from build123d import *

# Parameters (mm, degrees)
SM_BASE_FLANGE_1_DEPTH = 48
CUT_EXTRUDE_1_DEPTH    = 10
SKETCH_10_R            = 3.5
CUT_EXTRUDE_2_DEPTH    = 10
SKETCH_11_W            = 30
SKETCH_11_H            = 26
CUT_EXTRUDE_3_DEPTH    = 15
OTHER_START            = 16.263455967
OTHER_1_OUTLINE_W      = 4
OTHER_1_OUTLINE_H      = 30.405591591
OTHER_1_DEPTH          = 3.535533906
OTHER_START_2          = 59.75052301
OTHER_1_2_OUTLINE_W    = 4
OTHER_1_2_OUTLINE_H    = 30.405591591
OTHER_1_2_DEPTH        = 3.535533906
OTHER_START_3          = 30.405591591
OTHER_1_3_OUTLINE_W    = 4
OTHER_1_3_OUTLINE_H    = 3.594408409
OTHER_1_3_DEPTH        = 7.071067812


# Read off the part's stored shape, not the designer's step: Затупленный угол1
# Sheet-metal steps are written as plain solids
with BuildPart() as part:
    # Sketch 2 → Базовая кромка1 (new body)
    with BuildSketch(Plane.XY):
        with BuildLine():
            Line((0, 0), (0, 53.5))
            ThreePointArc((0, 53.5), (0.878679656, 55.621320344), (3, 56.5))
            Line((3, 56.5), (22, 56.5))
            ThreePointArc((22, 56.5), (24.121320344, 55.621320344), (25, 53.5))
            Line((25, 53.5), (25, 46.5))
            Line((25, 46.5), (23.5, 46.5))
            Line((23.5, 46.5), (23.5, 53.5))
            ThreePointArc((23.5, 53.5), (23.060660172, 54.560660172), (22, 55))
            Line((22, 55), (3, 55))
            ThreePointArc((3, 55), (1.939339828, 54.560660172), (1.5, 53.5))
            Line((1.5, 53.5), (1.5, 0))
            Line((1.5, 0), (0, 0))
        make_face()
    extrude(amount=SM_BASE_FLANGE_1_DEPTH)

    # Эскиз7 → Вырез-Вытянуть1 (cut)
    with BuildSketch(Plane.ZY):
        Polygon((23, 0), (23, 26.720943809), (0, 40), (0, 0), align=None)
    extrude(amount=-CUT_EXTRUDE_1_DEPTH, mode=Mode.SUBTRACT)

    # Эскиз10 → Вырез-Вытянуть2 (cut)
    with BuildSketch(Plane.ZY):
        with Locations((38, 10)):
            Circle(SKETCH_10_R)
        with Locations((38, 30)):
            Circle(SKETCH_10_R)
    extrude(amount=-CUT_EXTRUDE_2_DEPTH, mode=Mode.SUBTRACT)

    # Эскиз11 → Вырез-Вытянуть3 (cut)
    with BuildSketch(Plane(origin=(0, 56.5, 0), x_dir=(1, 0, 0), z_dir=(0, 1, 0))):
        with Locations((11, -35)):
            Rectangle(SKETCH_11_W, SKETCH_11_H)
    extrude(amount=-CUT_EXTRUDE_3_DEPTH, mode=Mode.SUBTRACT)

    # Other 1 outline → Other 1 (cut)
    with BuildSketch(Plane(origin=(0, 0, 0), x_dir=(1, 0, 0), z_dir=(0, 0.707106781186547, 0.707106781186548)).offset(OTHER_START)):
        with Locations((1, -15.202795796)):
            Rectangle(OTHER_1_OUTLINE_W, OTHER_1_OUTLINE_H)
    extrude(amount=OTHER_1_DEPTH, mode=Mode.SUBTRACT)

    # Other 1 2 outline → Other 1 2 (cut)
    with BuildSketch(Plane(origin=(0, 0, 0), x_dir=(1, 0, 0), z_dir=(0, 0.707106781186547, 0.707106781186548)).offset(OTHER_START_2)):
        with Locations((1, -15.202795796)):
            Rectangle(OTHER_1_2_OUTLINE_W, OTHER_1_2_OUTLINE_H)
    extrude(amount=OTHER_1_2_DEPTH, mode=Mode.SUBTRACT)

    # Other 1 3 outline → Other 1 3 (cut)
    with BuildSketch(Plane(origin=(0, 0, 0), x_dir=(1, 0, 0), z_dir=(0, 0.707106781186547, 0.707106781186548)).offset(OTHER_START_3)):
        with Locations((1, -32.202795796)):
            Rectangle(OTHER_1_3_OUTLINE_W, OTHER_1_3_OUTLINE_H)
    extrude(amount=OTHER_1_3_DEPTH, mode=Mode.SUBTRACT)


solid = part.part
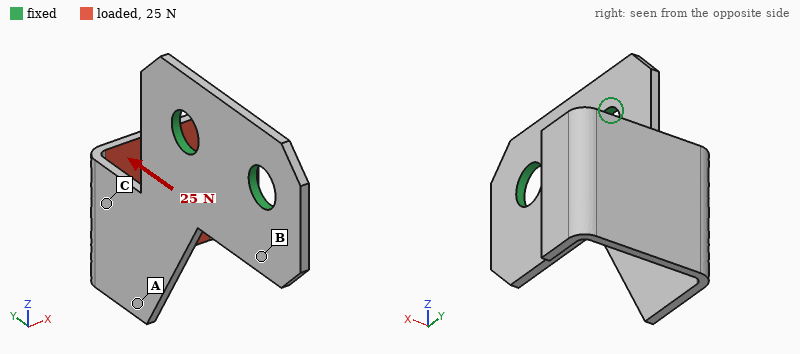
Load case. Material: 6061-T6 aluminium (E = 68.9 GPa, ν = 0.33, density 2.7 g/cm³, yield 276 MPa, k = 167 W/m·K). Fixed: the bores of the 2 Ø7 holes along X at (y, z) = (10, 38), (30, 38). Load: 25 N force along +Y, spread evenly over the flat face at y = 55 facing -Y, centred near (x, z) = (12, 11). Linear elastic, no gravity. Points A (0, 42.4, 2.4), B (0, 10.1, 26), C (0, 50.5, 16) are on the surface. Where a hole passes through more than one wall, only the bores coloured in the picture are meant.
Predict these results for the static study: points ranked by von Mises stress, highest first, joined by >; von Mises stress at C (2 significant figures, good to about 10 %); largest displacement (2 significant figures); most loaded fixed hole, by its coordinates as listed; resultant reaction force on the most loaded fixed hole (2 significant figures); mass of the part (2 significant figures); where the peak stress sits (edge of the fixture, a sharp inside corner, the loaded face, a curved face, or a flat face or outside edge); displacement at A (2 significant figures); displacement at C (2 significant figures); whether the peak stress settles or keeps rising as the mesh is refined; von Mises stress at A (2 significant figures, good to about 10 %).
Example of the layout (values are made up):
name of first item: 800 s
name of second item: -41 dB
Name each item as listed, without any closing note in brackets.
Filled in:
points ranked by von Mises stress, highest first, joined by >: C > A > B
von Mises stress at C: 34 MPa
largest displacement: 0.83 mm
most loaded fixed hole, by its coordinates as listed: (10, 38)
resultant reaction force on the most loaded fixed hole: 29 N
mass of the part: 8.5 g
where the peak stress sits: a sharp inside corner
displacement at A: 0.16 mm
displacement at C: 0.28 mm
whether the peak stress settles or keeps rising as the mesh is refined: keeps rising
von Mises stress at A: 22 MPa
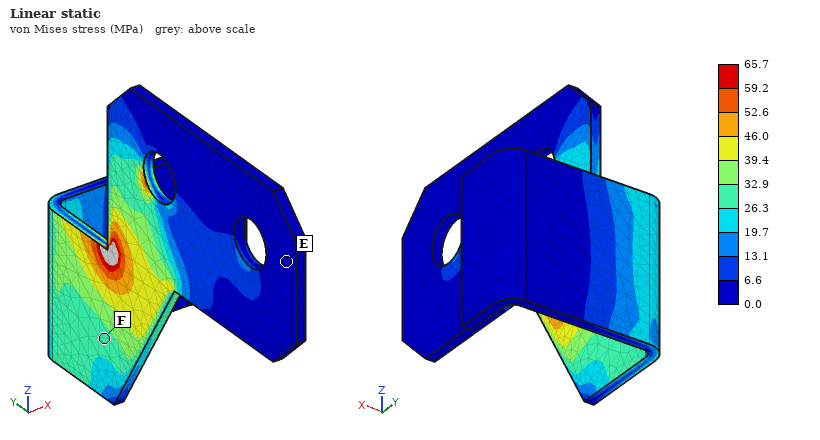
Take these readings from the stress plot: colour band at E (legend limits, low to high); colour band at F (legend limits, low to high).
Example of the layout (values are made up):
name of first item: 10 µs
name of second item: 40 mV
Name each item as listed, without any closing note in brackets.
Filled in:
colour band at E: 0.0 to 6.6 MPa
colour band at F: 26.3 to 32.9 MPa
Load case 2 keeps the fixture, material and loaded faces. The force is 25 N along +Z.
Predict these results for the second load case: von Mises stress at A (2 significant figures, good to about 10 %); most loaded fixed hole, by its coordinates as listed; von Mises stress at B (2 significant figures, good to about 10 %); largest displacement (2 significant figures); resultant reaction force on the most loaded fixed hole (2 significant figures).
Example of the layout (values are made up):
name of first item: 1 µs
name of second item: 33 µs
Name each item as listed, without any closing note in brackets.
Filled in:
von Mises stress at A: 11 MPa
most loaded fixed hole, by its coordinates as listed: (30, 38)
von Mises stress at B: 6.4 MPa
largest displacement: 0.90 mm
resultant reaction force on the most loaded fixed hole: 46 N
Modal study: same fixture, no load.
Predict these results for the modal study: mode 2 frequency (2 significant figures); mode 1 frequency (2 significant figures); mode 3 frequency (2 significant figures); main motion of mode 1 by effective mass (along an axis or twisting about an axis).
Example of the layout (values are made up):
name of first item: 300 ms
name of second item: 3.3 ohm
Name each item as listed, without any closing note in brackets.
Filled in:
mode 2 frequency: 590 Hz
mode 1 frequency: 340 Hz
mode 3 frequency: 1100 Hz
main motion of mode 1 by effective mass: along X
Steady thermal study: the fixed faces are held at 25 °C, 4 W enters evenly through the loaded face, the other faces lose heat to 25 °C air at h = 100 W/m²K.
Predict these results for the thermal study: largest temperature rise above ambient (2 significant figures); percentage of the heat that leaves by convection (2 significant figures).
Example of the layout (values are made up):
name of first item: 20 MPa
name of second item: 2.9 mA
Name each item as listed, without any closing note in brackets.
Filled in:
largest temperature rise above ambient: 17 K
percentage of the heat that leaves by convection: 70 %
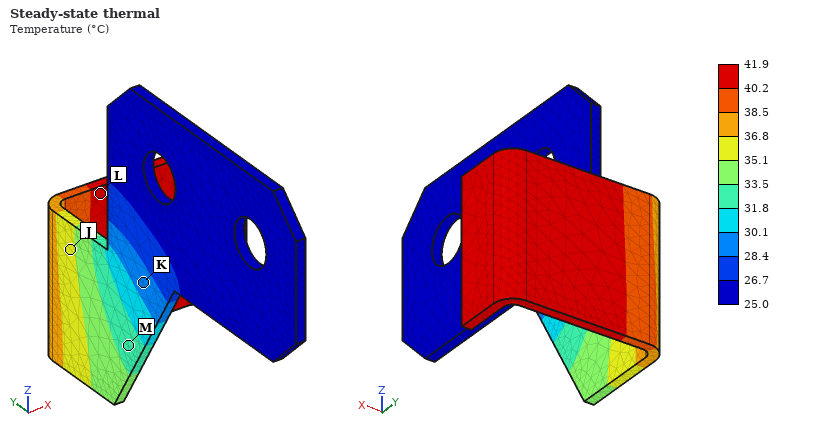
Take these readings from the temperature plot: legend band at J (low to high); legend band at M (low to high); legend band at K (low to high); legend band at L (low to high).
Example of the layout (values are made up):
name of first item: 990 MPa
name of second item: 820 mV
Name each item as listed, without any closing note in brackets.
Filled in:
legend band at J: 35.1 to 36.8 °C
legend band at M: 31.8 to 33.5 °C
legend band at K: 28.4 to 30.1 °C
legend band at L: 40.2 to 41.9 °C
